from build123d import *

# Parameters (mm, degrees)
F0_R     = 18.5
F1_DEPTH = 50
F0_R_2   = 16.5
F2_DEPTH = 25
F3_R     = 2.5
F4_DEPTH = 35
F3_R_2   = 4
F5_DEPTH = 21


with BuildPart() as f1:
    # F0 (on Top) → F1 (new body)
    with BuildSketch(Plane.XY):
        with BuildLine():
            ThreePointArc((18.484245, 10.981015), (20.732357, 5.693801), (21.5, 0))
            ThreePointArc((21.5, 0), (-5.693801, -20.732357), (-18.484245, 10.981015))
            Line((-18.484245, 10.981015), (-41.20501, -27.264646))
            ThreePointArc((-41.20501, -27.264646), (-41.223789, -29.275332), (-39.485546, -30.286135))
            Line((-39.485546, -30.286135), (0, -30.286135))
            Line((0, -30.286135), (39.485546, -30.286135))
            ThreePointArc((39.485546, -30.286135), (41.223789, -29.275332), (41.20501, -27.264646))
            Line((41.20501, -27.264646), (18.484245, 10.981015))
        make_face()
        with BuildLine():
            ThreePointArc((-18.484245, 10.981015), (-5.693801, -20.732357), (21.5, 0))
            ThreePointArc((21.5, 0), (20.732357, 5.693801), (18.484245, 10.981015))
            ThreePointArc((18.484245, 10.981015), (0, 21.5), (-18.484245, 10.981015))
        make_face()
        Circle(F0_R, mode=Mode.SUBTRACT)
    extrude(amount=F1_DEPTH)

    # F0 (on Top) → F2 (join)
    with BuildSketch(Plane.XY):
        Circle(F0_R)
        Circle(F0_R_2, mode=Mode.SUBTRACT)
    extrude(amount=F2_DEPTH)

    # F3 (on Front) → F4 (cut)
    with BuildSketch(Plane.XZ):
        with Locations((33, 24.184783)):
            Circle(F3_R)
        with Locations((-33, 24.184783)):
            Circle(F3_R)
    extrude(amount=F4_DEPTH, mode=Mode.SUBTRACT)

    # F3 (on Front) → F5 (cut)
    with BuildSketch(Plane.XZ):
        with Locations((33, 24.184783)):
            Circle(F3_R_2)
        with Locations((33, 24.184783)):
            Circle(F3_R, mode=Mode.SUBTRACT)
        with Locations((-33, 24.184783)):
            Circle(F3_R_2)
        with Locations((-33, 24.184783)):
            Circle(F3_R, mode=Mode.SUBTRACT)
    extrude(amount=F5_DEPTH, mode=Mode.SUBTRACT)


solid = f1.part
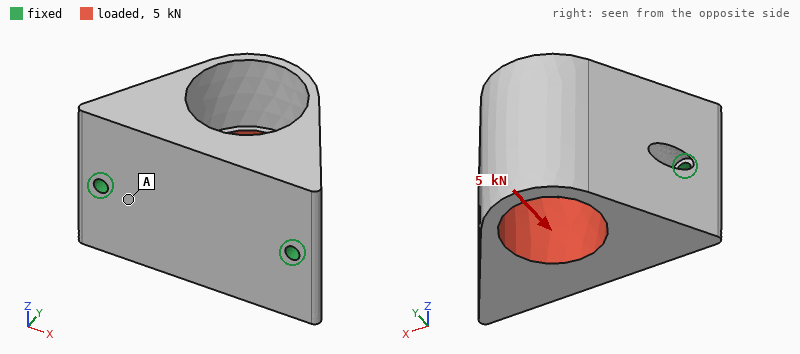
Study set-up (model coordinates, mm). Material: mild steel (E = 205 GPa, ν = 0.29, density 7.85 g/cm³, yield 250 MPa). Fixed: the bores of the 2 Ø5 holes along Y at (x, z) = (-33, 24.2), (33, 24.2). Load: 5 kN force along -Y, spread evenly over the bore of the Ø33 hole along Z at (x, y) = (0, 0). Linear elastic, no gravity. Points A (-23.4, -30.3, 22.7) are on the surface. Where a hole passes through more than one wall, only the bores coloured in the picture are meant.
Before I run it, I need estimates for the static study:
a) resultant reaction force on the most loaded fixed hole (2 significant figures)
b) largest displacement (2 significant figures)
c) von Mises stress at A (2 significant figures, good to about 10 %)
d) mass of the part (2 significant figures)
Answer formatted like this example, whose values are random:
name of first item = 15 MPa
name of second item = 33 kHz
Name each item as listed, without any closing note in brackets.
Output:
resultant reaction force on the most loaded fixed hole = 2.7 kN
largest displacement = 24 µm
von Mises stress at A = 11 MPa
mass of the part = 710 g
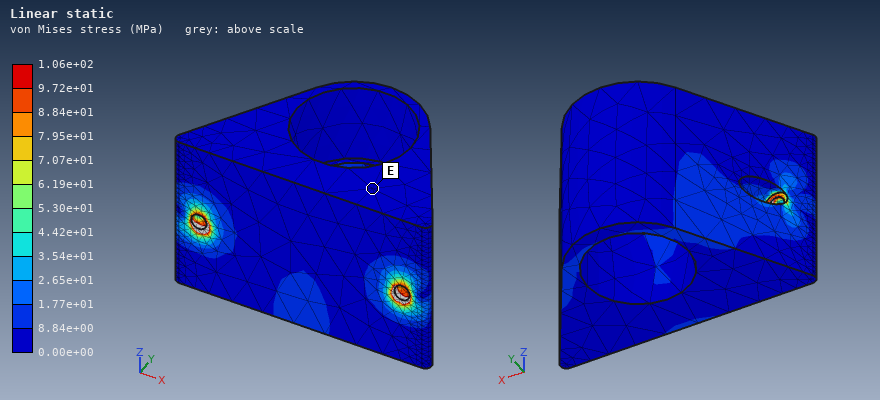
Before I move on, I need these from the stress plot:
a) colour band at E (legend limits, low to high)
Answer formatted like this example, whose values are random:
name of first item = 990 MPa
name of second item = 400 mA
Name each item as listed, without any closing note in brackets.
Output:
colour band at E = 0.00e+00 to 8.84e+00 MPa
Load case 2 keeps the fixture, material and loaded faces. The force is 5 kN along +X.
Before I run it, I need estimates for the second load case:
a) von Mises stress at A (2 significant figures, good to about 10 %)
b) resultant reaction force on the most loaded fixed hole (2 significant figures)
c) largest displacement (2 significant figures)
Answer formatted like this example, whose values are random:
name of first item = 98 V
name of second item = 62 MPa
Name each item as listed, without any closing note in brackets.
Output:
von Mises stress at A = 6.2 MPa
resultant reaction force on the most loaded fixed hole = 3.2 kN
largest displacement = 10 µm
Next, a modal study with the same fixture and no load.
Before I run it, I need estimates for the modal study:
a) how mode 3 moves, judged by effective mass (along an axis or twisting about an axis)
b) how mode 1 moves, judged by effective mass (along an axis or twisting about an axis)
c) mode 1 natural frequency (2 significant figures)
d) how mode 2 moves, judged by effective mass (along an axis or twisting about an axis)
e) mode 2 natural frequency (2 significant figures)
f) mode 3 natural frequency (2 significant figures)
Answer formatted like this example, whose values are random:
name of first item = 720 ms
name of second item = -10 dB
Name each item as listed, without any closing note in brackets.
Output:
how mode 3 moves, judged by effective mass = along X
how mode 1 moves, judged by effective mass = along Z
mode 1 natural frequency = 3100 Hz
how mode 2 moves, judged by effective mass = along Y
mode 2 natural frequency = 7700 Hz
mode 3 natural frequency = 8700 Hz
